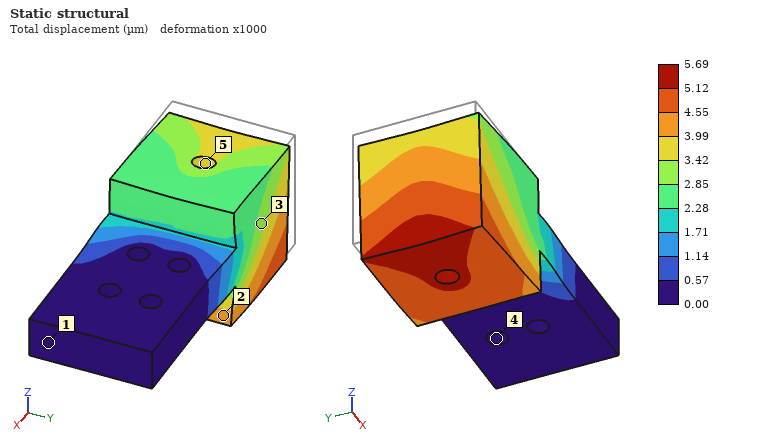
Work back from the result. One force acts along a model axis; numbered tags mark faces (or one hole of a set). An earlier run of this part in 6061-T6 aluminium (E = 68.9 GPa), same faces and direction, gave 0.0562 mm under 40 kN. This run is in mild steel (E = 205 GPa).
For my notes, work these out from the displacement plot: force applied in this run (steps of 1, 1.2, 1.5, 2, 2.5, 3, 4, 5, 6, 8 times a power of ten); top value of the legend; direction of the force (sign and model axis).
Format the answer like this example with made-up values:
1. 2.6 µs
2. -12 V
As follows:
1. 12 kN
2. 5.69 µm
3. +X
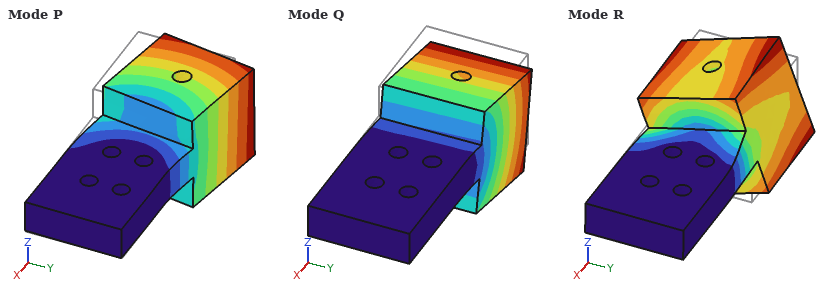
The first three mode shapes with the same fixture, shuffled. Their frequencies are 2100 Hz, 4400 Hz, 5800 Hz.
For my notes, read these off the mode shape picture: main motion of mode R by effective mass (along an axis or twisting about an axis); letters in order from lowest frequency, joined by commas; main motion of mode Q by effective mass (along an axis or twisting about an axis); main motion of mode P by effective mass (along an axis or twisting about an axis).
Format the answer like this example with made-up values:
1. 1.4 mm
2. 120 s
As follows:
1. twisting about X
2. Q, P, R
3. along Z
4. along Y
